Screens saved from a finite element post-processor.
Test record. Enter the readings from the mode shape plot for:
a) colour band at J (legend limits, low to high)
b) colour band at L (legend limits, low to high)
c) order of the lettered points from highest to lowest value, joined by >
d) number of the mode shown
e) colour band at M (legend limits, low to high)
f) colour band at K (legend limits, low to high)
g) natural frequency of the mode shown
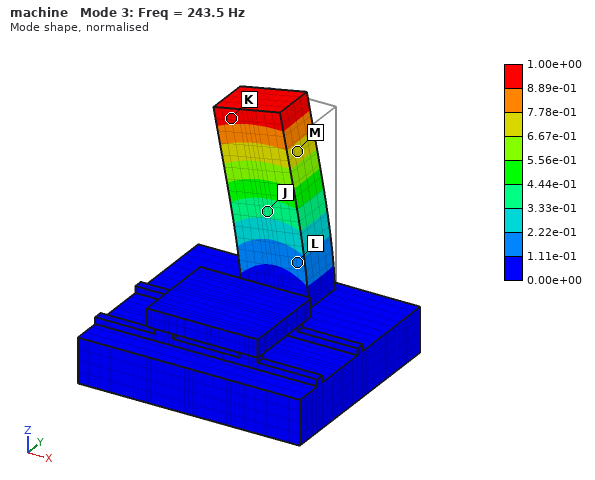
3.33e-01 to 4.44e-01
1.11e-01 to 2.22e-01
K > M > J > L
3
6.67e-01 to 7.78e-01
8.89e-01 to 1.00e+00
243.5 Hz
